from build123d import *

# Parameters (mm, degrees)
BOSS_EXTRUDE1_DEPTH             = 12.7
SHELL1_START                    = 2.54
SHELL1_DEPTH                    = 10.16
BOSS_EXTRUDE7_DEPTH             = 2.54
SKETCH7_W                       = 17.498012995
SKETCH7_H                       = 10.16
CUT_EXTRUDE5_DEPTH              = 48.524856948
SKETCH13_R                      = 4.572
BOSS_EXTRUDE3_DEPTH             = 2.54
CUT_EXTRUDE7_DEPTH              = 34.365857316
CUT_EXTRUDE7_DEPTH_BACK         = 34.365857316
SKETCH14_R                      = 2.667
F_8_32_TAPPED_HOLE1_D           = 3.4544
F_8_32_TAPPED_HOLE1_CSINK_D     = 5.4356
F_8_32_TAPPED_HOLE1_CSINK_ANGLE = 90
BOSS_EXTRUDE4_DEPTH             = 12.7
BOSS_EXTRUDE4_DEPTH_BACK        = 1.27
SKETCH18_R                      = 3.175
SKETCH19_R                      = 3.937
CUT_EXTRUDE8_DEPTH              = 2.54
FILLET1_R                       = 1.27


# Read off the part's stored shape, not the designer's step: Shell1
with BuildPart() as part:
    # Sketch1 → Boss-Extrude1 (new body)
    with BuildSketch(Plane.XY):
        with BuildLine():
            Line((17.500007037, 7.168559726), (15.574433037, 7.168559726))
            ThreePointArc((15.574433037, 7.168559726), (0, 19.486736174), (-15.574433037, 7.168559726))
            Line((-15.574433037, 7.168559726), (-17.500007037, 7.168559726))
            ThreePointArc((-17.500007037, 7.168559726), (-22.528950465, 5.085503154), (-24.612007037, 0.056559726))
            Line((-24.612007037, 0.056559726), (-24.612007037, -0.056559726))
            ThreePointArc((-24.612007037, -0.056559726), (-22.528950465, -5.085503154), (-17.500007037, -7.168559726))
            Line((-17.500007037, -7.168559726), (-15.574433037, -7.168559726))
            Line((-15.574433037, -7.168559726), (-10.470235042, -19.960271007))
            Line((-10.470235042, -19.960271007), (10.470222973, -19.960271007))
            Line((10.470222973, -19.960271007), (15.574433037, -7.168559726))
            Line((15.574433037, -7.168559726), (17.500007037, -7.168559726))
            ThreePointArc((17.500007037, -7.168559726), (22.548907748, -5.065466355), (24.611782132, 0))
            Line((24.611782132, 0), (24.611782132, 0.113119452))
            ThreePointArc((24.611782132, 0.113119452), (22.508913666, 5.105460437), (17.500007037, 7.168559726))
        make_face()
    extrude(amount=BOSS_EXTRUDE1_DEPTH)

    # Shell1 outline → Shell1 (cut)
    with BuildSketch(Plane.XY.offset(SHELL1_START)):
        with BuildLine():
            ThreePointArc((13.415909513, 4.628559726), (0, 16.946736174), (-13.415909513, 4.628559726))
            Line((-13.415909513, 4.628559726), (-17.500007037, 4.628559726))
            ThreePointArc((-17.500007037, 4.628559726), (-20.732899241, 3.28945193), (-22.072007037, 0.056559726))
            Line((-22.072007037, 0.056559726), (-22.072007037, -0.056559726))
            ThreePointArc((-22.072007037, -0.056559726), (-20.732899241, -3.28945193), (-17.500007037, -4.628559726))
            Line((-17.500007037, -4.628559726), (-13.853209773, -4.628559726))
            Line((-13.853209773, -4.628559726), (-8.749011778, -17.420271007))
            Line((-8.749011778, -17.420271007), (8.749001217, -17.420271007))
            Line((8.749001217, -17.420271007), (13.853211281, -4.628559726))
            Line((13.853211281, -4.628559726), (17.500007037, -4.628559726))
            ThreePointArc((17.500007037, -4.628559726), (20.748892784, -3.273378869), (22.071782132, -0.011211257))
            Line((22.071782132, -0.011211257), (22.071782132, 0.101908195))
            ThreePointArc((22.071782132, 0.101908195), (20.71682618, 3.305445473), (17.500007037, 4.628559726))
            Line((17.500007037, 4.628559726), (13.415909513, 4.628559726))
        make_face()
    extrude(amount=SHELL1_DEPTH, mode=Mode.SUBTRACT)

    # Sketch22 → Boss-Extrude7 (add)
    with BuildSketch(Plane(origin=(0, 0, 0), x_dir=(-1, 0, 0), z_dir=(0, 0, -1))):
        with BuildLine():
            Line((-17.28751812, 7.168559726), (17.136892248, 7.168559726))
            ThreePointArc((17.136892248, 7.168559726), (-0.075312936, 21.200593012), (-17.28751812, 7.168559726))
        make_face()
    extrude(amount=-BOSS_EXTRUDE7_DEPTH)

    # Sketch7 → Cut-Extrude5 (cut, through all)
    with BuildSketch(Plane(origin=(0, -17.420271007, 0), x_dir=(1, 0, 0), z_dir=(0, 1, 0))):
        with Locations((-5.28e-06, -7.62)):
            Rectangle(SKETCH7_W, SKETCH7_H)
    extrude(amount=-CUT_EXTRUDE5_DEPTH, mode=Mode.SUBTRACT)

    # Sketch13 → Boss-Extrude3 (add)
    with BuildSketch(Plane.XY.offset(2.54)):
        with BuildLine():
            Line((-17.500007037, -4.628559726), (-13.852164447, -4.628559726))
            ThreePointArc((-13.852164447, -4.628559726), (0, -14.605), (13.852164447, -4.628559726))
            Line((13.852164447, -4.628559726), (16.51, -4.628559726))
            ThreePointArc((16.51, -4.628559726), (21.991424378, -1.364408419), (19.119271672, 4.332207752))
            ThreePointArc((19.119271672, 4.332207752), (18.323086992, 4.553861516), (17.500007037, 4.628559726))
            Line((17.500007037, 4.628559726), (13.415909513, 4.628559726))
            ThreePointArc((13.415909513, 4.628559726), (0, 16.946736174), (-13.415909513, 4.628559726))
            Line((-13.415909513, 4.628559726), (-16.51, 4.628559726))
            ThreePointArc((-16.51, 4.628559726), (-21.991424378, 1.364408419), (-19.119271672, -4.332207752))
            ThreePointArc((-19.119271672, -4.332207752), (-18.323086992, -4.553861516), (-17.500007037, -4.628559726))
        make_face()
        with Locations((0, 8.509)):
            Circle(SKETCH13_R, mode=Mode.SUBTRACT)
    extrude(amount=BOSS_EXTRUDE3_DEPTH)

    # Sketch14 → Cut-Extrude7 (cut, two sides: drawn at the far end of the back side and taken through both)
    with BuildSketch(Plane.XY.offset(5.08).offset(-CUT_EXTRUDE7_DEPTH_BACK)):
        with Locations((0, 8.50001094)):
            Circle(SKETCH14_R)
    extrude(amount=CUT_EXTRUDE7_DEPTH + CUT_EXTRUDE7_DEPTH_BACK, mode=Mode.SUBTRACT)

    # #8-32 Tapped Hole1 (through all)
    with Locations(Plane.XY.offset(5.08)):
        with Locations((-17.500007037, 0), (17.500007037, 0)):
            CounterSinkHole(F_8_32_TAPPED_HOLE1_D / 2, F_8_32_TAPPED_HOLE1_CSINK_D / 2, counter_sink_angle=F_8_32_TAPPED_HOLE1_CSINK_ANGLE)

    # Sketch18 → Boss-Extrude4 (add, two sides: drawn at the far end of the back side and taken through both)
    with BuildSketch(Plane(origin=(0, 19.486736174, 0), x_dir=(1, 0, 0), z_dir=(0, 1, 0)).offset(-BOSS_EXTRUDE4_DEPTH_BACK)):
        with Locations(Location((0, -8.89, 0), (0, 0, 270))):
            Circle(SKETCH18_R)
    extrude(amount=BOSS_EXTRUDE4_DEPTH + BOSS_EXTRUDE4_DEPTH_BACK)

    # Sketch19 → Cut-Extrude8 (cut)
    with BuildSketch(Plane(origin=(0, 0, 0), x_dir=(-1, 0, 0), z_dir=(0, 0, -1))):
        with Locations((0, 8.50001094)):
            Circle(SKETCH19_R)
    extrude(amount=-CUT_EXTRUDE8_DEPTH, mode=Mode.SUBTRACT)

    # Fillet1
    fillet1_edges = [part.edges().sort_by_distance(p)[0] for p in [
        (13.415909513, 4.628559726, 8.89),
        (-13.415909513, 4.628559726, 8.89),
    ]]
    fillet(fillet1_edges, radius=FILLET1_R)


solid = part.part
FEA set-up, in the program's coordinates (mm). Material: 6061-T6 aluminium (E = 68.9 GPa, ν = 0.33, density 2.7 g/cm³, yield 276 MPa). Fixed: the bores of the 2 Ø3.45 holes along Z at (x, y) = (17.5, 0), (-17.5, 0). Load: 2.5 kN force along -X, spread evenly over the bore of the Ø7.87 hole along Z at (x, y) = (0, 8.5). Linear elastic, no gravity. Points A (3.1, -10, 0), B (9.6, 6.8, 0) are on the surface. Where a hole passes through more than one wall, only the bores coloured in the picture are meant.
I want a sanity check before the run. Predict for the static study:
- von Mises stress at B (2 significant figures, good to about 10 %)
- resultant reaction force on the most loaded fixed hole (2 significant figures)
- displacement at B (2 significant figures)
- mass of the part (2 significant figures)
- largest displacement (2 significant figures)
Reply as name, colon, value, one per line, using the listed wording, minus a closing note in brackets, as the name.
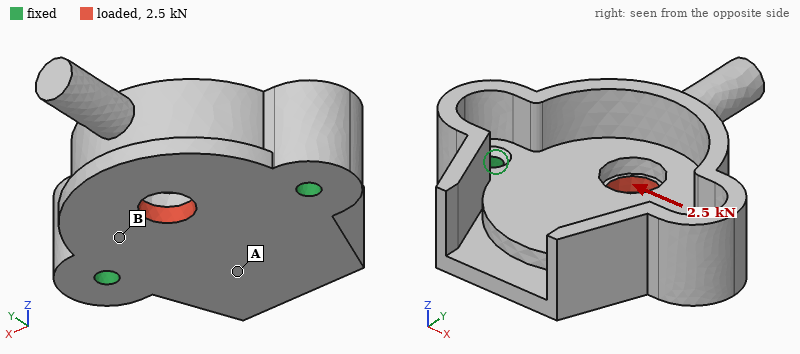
von Mises stress at B: 36 MPa
resultant reaction force on the most loaded fixed hole: 1.4 kN
displacement at B: 5.3 µm
mass of the part: 23 g
largest displacement: 11 µm
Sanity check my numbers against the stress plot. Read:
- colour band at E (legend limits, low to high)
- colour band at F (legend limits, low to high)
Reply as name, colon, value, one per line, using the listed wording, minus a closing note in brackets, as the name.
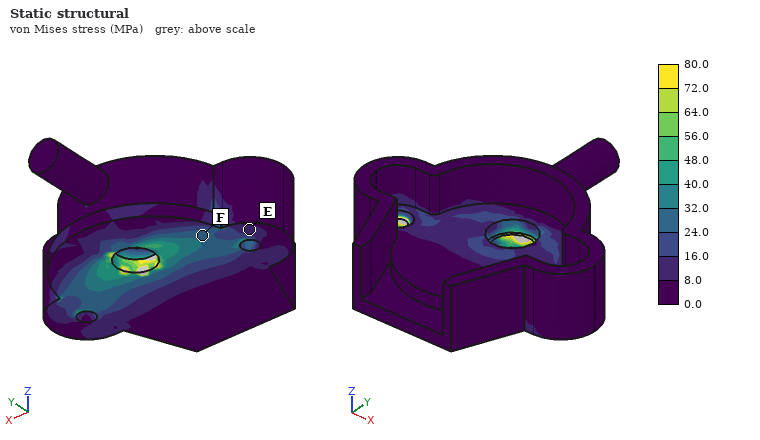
colour band at E: 8.0 to 16.0 MPa
colour band at F: 24.0 to 32.0 MPa
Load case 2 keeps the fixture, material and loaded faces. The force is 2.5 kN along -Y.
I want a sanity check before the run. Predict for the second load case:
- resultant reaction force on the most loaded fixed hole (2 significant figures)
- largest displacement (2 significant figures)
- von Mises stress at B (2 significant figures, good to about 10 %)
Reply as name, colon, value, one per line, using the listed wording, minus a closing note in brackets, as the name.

resultant reaction force on the most loaded fixed hole: 1.3 kN
largest displacement: 41 µm
von Mises stress at B: 23 MPa
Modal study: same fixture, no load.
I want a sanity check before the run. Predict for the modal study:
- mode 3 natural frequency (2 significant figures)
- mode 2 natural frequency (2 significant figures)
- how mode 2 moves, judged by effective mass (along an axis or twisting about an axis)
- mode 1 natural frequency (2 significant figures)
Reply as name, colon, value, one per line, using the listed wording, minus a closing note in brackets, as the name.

mode 3 natural frequency: 13 kHz
mode 2 natural frequency: 9000 Hz
how mode 2 moves, judged by effective mass: along Z
mode 1 natural frequency: 5500 Hz
